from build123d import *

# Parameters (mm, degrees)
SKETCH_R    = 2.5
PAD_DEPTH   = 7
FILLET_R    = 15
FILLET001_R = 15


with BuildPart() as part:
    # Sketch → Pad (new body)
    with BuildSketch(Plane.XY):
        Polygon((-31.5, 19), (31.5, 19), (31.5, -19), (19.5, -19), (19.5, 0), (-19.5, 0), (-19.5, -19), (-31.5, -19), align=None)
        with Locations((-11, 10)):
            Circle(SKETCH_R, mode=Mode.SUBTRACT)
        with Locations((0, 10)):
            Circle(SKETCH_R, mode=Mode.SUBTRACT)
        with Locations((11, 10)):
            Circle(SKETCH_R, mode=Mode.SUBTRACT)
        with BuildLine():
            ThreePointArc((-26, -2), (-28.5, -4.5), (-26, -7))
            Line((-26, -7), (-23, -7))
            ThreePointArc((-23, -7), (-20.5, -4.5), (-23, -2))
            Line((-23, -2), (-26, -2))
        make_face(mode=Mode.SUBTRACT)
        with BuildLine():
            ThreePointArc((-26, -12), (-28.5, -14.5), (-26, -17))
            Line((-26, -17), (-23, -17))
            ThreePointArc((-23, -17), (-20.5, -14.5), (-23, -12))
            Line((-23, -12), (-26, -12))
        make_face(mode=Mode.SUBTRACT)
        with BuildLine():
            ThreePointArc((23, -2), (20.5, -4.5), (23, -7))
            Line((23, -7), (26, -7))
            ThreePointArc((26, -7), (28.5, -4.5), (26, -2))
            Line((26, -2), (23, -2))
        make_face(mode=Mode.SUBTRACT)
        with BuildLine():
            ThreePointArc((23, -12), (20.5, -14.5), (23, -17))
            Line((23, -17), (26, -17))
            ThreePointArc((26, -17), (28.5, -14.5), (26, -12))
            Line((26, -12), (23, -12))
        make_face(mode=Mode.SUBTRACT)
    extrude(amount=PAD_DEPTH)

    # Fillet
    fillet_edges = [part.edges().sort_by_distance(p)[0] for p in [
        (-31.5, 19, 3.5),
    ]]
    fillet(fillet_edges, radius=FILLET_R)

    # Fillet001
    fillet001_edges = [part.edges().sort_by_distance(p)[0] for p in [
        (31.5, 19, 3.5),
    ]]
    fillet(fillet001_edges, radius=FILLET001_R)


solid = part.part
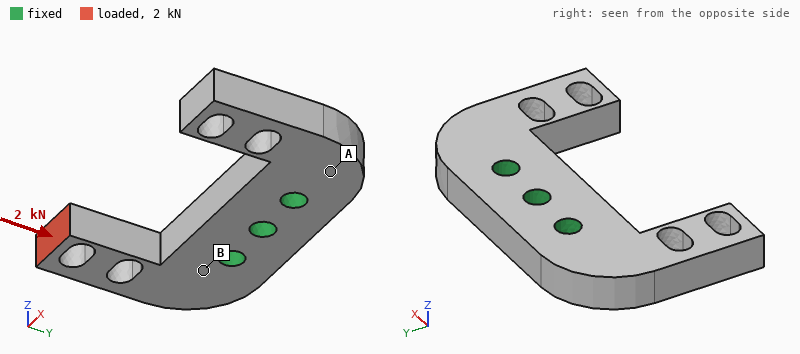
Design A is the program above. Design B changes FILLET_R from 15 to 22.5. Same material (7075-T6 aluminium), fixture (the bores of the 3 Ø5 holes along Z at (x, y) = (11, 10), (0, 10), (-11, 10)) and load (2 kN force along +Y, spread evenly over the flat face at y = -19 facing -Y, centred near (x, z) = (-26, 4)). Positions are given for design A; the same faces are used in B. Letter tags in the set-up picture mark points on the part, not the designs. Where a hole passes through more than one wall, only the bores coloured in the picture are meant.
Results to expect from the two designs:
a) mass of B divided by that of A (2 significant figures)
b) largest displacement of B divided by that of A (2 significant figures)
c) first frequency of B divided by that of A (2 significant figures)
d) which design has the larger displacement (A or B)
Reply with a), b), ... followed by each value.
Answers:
a) 0.96
b) 1.1
c) 0.98
d) B
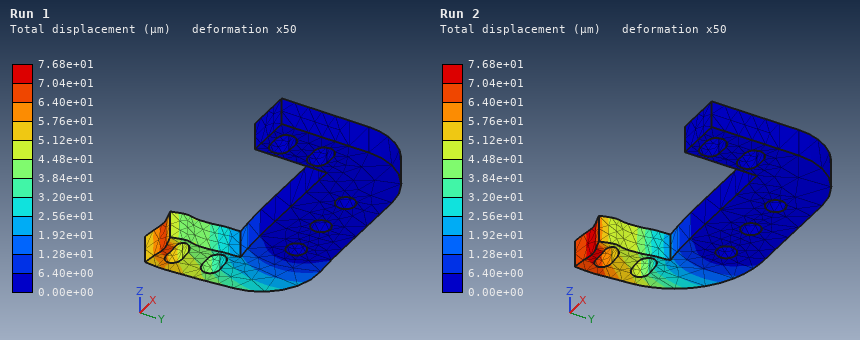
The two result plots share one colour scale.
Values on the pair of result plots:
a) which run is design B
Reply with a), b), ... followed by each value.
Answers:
a) Run 2
